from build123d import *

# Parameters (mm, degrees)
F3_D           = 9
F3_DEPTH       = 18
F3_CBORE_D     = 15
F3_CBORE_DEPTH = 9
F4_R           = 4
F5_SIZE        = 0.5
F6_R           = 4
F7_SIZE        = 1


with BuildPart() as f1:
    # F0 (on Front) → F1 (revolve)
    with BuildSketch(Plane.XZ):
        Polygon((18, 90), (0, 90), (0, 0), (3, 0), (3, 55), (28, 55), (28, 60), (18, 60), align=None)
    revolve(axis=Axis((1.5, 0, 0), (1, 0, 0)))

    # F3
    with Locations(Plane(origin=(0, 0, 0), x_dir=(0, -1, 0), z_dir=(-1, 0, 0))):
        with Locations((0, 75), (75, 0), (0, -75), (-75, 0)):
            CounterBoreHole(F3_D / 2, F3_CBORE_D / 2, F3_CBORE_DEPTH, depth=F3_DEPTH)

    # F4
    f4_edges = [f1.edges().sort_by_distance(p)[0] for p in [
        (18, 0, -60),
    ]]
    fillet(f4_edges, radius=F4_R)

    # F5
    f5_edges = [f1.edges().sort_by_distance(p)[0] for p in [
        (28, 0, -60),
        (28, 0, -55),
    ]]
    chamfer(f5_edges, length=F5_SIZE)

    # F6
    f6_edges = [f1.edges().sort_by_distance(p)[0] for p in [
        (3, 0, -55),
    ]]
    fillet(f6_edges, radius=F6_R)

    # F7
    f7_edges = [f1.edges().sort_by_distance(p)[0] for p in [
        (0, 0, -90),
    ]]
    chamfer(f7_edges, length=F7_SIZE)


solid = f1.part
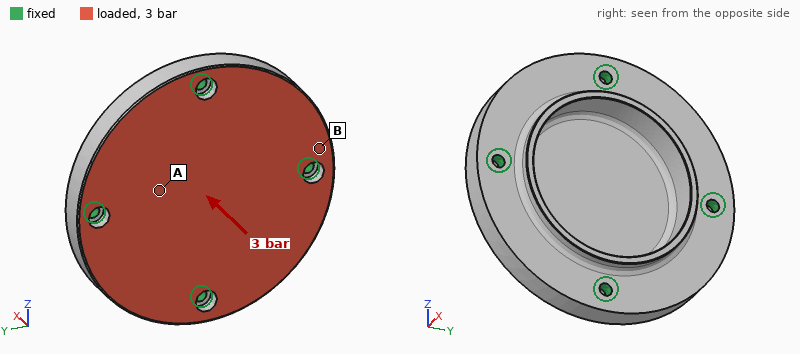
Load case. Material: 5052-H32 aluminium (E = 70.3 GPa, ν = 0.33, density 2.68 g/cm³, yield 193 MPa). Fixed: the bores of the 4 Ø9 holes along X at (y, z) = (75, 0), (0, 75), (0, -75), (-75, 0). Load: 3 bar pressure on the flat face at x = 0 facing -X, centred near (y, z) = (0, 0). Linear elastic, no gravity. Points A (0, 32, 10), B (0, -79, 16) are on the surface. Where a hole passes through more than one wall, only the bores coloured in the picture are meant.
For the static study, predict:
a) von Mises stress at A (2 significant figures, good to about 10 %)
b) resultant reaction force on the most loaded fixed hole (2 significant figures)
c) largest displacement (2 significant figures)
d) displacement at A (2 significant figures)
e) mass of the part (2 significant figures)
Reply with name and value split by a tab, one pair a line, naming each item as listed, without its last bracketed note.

von Mises stress at A	22 MPa
resultant reaction force on the most loaded fixed hole	2.0 kN
largest displacement	0.24 mm
displacement at A	0.097 mm
mass of the part	880 g
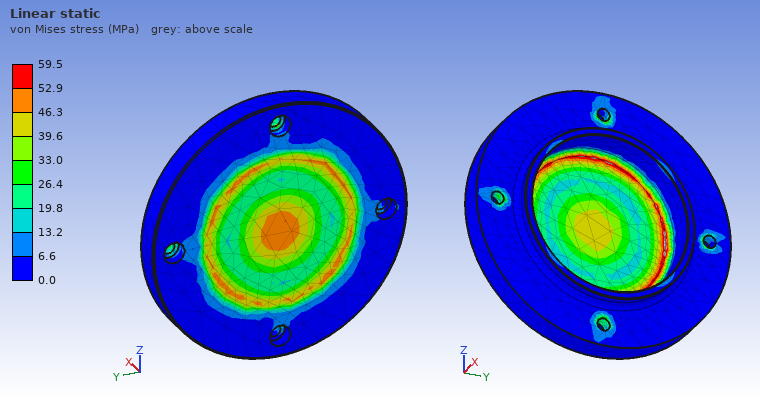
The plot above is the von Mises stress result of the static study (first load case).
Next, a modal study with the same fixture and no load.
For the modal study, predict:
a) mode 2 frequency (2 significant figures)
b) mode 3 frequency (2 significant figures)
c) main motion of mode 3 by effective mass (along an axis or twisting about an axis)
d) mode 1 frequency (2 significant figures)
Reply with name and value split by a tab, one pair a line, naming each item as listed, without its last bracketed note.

mode 2 frequency	4000 Hz
mode 3 frequency	4800 Hz
main motion of mode 3 by effective mass	twisting about Y
mode 1 frequency	2500 Hz
